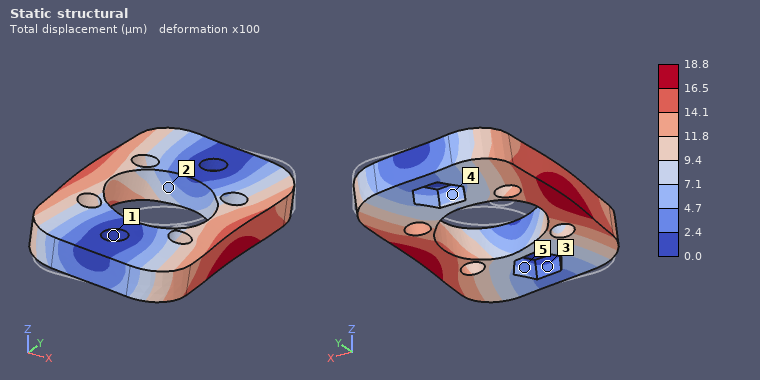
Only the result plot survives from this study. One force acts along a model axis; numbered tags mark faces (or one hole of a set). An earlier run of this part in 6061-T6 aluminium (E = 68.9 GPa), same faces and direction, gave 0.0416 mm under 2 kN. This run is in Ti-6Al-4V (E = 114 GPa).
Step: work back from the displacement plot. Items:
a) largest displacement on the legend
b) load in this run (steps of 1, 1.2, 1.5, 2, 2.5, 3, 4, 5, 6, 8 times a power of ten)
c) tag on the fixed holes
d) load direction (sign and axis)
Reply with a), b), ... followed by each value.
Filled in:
a) 18.8 µm
b) 1.5 kN
c) 1
d) -X
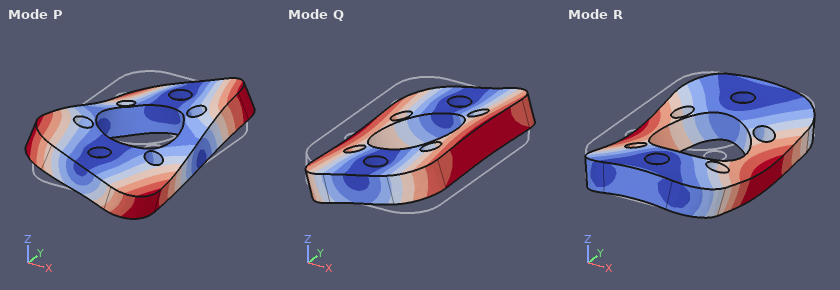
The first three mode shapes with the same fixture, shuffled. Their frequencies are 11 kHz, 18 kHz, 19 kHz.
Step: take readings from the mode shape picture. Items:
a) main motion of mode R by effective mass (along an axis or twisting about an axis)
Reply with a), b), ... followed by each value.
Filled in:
a) along Z
